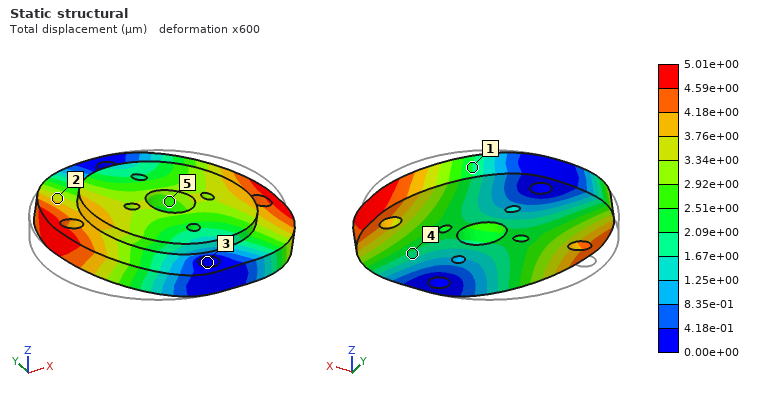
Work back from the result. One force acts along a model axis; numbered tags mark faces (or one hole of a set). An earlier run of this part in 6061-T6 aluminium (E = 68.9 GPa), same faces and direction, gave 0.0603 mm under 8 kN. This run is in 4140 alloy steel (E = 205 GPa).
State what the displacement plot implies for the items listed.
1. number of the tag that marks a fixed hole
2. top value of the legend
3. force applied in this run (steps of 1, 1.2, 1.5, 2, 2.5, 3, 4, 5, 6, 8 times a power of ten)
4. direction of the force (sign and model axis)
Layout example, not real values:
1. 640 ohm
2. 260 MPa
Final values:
1. 3
2. 5.01e+00 µm
3. 2 kN
4. +X
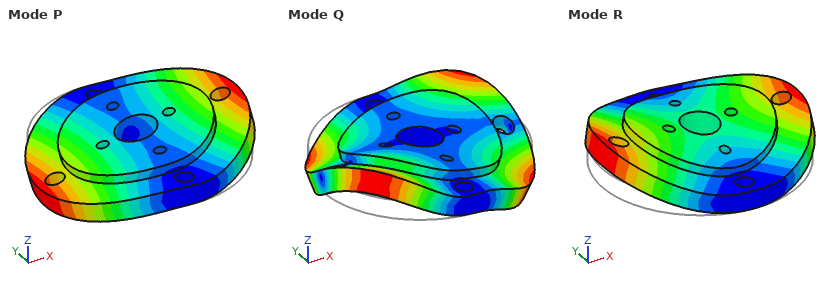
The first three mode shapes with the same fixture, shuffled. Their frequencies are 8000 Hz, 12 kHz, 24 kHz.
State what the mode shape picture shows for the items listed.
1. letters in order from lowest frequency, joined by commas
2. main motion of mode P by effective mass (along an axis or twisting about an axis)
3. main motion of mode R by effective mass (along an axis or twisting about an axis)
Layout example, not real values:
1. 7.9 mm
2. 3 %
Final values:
1. P, R, Q
2. twisting about Y
3. along Z
